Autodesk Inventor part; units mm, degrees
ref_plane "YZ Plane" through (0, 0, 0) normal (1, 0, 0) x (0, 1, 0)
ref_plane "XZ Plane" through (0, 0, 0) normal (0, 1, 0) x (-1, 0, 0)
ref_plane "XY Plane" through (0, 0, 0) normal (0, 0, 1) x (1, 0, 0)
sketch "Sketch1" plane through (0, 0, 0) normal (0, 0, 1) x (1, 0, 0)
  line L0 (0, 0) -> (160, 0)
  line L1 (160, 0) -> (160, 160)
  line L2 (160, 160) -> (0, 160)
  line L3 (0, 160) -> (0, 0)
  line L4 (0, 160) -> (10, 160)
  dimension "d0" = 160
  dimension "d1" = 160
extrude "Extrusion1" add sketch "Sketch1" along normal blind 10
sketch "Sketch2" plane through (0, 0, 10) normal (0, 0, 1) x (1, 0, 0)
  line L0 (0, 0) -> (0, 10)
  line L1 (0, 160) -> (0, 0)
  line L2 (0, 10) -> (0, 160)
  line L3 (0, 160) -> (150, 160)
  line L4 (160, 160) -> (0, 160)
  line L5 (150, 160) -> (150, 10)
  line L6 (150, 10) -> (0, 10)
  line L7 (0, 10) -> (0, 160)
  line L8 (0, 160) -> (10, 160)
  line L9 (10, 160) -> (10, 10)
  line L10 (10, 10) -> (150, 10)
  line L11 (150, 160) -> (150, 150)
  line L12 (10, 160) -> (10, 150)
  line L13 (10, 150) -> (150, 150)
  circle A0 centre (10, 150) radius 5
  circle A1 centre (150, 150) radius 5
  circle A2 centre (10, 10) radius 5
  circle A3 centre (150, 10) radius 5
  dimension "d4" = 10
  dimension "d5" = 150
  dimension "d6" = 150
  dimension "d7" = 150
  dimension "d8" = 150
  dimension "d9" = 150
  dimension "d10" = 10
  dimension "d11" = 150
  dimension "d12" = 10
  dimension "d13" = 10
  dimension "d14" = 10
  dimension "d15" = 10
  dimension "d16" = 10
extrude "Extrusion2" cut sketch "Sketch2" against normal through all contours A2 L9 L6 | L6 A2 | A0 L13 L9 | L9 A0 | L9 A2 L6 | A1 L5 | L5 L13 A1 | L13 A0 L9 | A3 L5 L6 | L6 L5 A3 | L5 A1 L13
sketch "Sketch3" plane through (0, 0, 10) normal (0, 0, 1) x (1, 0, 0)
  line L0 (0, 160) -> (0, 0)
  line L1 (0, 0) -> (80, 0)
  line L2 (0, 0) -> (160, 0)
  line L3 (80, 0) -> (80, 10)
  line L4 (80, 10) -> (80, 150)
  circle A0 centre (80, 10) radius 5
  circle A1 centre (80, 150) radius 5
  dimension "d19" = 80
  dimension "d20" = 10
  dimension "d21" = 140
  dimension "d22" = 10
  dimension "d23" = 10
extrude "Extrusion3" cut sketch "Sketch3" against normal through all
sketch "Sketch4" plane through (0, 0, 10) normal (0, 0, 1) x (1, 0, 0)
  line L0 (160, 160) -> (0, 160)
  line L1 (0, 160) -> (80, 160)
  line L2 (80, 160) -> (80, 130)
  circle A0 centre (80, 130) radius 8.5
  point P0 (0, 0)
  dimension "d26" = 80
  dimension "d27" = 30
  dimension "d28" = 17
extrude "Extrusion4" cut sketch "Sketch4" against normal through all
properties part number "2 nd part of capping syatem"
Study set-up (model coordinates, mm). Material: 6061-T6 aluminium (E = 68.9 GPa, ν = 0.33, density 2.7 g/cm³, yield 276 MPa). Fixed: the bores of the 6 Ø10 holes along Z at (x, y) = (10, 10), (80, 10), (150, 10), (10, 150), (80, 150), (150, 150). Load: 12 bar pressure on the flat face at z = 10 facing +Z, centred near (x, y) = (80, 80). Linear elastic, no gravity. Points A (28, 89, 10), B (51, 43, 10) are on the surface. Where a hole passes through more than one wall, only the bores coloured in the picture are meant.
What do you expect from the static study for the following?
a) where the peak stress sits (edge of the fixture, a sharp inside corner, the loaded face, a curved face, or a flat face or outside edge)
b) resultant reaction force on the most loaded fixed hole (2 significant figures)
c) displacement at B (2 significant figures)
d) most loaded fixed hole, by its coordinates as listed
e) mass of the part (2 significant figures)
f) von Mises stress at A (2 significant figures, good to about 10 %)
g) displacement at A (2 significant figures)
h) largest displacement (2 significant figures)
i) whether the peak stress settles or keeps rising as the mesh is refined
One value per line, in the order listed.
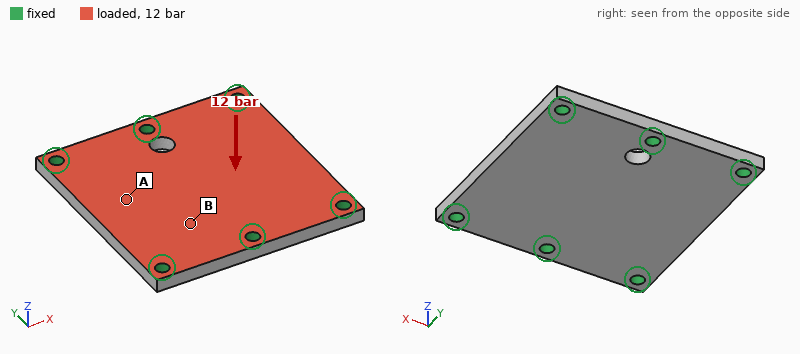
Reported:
edge of the fixture
6.9 kN
0.16 mm
(80, 10)
670 g
55 MPa
0.24 mm
0.26 mm
keeps rising
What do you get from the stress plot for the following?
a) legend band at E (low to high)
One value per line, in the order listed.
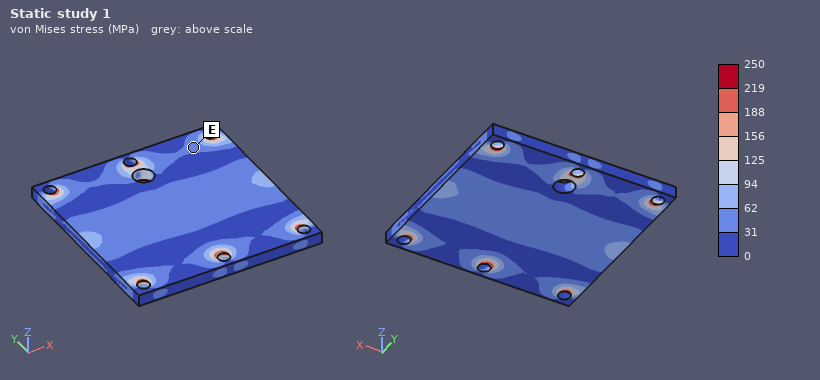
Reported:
31 to 62 MPa
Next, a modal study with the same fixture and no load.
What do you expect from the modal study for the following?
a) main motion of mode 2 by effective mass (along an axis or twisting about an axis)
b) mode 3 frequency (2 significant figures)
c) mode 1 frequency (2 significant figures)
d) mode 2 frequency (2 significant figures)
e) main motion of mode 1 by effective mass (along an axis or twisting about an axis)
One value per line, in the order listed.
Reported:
twisting about Y
4500 Hz
2400 Hz
2900 Hz
along Z
